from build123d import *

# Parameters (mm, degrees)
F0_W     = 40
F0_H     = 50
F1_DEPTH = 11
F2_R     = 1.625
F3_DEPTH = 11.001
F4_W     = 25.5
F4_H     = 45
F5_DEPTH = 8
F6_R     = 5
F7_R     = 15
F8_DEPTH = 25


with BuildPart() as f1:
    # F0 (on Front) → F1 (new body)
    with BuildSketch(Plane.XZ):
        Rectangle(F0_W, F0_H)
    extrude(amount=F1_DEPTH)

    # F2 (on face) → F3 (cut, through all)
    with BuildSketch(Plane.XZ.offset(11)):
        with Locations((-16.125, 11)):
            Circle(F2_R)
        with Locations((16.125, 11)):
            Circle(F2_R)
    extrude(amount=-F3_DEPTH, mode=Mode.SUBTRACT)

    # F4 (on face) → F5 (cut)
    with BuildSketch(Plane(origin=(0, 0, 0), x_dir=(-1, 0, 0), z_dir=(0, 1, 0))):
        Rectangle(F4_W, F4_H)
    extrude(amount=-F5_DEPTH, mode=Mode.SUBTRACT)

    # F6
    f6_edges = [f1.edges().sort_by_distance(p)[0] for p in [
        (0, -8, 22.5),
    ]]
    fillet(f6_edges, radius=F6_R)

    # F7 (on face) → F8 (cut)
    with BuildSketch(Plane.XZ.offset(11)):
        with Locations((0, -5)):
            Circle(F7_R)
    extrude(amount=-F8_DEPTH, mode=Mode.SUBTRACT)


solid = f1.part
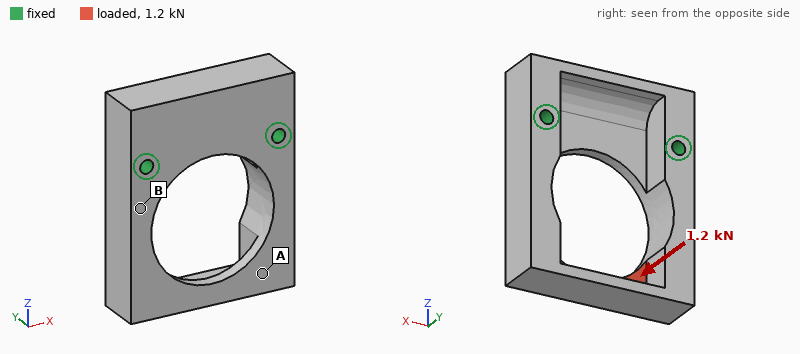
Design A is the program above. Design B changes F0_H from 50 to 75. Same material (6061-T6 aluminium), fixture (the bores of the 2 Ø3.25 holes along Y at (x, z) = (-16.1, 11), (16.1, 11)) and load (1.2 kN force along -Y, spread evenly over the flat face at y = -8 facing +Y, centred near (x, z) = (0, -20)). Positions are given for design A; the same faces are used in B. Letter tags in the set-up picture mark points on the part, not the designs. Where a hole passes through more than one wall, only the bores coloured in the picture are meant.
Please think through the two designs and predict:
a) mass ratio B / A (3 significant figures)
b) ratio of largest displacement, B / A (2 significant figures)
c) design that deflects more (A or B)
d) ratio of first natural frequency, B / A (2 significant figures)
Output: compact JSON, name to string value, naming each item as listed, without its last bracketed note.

{"mass ratio B / A": "2.07", "ratio of largest displacement, B / A": "1.3", "design that deflects more": "B", "ratio of first natural frequency, B / A": "0.45"}
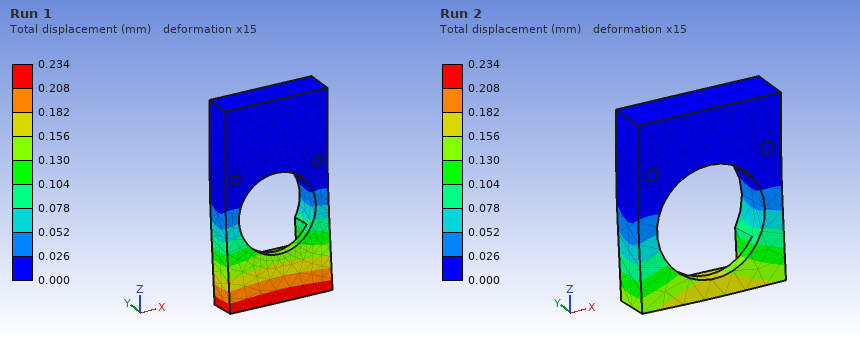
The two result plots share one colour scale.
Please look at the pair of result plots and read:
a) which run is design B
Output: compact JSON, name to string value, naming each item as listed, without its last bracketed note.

{"which run is design B": "Run 1"}
